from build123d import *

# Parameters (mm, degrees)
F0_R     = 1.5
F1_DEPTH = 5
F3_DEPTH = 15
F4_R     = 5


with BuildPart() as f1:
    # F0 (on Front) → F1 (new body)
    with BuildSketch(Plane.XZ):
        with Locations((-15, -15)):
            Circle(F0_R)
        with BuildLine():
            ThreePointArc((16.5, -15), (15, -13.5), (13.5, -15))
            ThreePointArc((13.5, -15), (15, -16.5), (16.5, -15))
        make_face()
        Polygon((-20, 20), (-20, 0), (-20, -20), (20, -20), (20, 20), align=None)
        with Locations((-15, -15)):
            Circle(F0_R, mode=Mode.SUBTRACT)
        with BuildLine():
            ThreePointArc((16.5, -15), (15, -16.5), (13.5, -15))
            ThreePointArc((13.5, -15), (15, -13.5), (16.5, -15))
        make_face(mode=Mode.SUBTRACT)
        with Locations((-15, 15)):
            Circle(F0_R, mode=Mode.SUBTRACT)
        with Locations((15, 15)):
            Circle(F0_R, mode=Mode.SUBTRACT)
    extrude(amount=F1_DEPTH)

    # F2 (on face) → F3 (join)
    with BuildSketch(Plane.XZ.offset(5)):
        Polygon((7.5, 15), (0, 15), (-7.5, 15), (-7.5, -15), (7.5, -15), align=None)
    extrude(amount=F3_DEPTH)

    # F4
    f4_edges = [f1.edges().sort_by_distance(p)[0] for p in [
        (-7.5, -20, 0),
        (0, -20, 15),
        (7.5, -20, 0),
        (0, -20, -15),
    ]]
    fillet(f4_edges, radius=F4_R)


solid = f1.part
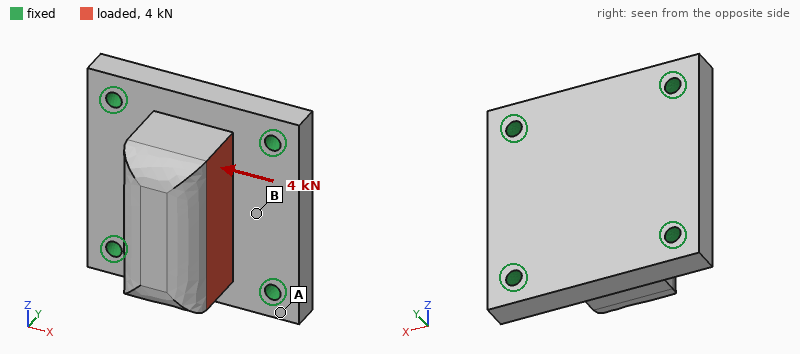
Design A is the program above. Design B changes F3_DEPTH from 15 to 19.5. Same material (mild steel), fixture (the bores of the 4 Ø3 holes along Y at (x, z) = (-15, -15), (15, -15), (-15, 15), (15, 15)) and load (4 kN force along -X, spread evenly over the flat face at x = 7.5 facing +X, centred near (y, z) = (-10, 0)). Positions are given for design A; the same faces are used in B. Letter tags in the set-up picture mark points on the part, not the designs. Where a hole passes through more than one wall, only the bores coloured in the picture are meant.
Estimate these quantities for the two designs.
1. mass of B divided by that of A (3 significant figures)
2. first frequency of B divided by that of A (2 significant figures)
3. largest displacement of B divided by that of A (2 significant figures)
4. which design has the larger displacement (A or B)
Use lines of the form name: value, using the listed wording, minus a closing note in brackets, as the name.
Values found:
mass of B divided by that of A: 1.14
first frequency of B divided by that of A: 0.83
largest displacement of B divided by that of A: 1.6
which design has the larger displacement: B
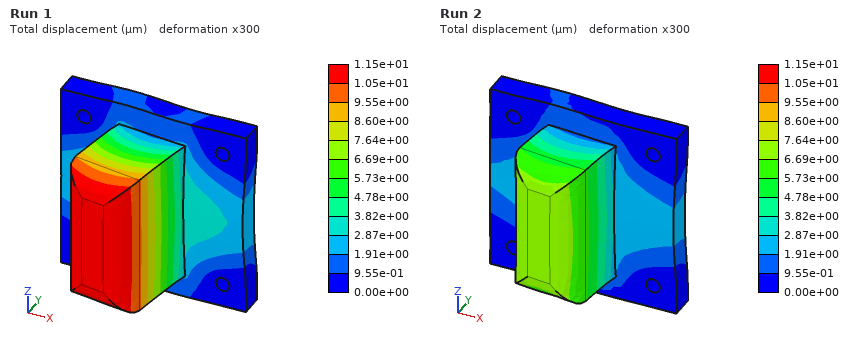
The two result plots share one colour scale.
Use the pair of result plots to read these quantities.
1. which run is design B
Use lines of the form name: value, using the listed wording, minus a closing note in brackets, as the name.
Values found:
which run is design B: Run 1
